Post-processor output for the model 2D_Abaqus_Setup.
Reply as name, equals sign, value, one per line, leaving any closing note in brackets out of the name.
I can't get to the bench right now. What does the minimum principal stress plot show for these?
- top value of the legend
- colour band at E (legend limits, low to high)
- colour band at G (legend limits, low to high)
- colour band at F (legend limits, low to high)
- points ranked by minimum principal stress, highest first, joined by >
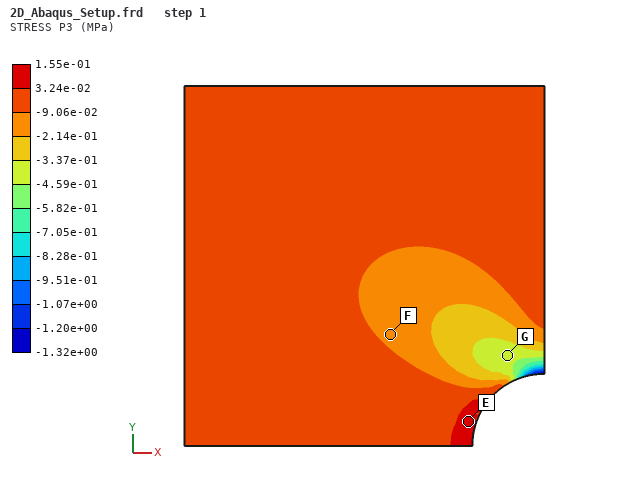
top value of the legend = 1.55e-01 MPa
colour band at E = 3.24e-02 to 1.55e-01 MPa
colour band at G = -4.59e-01 to -3.37e-01 MPa
colour band at F = -2.14e-01 to -9.06e-02 MPa
points ranked by minimum principal stress, highest first, joined by > = E > F > G
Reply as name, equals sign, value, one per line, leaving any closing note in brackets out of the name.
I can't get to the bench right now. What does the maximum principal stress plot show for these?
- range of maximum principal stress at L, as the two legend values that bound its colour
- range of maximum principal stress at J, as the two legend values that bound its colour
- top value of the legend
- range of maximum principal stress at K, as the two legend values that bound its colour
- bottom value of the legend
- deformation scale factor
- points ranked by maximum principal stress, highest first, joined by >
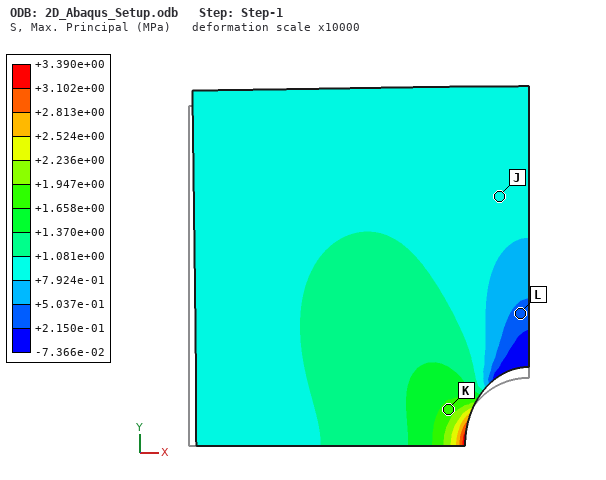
range of maximum principal stress at L, as the two legend values that bound its colour = +2.150e-01 to +5.037e-01 MPa
range of maximum principal stress at J, as the two legend values that bound its colour = +7.924e-01 to +1.081e+00 MPa
top value of the legend = +3.390e+00 MPa
range of maximum principal stress at K, as the two legend values that bound its colour = +1.658e+00 to +1.947e+00 MPa
bottom value of the legend = -7.366e-02 MPa
deformation scale factor = 10000
points ranked by maximum principal stress, highest first, joined by > = K > J > L
